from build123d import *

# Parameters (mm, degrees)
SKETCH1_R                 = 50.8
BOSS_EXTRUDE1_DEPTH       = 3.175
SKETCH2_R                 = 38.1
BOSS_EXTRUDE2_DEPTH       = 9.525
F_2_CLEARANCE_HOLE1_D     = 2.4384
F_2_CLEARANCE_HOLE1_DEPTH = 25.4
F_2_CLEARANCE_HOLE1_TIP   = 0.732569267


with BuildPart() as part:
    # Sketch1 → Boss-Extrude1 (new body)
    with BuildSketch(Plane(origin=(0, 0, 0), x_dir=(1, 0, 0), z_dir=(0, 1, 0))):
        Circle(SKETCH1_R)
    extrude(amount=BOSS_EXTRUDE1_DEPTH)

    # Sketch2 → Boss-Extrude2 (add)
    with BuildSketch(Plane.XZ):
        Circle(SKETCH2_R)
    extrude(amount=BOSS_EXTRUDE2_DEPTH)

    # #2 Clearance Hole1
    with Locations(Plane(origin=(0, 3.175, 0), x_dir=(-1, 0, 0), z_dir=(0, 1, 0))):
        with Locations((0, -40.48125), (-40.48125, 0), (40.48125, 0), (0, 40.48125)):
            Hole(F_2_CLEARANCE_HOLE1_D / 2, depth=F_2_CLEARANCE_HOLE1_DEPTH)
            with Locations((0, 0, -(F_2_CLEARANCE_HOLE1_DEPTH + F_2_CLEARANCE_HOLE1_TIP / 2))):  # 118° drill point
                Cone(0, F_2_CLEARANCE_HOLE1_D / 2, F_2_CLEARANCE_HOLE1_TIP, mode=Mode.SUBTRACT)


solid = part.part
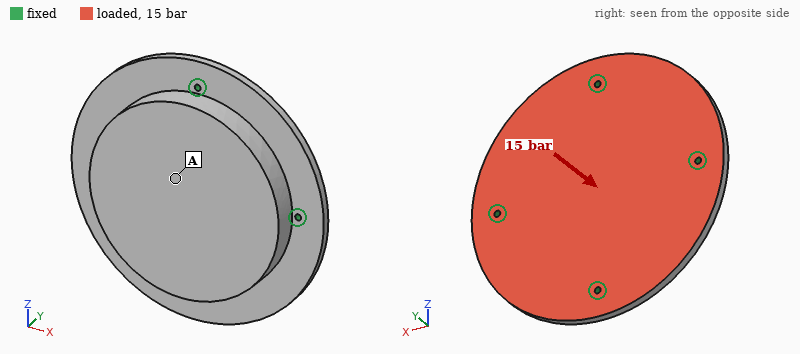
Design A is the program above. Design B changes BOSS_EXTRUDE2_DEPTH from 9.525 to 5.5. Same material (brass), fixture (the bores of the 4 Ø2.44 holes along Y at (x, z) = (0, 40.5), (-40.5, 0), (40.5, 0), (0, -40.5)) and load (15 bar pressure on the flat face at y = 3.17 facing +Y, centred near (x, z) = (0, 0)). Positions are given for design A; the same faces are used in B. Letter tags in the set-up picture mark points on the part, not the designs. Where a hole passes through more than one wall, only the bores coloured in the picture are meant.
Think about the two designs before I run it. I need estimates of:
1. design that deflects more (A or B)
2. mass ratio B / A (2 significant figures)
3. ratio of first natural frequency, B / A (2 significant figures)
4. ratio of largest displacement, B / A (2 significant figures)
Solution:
B
0.73
0.89
1.4
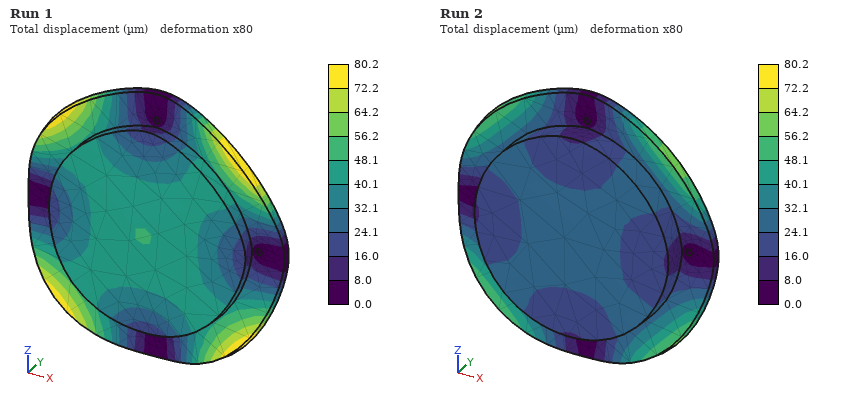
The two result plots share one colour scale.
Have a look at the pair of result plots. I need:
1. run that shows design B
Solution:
Run 1
